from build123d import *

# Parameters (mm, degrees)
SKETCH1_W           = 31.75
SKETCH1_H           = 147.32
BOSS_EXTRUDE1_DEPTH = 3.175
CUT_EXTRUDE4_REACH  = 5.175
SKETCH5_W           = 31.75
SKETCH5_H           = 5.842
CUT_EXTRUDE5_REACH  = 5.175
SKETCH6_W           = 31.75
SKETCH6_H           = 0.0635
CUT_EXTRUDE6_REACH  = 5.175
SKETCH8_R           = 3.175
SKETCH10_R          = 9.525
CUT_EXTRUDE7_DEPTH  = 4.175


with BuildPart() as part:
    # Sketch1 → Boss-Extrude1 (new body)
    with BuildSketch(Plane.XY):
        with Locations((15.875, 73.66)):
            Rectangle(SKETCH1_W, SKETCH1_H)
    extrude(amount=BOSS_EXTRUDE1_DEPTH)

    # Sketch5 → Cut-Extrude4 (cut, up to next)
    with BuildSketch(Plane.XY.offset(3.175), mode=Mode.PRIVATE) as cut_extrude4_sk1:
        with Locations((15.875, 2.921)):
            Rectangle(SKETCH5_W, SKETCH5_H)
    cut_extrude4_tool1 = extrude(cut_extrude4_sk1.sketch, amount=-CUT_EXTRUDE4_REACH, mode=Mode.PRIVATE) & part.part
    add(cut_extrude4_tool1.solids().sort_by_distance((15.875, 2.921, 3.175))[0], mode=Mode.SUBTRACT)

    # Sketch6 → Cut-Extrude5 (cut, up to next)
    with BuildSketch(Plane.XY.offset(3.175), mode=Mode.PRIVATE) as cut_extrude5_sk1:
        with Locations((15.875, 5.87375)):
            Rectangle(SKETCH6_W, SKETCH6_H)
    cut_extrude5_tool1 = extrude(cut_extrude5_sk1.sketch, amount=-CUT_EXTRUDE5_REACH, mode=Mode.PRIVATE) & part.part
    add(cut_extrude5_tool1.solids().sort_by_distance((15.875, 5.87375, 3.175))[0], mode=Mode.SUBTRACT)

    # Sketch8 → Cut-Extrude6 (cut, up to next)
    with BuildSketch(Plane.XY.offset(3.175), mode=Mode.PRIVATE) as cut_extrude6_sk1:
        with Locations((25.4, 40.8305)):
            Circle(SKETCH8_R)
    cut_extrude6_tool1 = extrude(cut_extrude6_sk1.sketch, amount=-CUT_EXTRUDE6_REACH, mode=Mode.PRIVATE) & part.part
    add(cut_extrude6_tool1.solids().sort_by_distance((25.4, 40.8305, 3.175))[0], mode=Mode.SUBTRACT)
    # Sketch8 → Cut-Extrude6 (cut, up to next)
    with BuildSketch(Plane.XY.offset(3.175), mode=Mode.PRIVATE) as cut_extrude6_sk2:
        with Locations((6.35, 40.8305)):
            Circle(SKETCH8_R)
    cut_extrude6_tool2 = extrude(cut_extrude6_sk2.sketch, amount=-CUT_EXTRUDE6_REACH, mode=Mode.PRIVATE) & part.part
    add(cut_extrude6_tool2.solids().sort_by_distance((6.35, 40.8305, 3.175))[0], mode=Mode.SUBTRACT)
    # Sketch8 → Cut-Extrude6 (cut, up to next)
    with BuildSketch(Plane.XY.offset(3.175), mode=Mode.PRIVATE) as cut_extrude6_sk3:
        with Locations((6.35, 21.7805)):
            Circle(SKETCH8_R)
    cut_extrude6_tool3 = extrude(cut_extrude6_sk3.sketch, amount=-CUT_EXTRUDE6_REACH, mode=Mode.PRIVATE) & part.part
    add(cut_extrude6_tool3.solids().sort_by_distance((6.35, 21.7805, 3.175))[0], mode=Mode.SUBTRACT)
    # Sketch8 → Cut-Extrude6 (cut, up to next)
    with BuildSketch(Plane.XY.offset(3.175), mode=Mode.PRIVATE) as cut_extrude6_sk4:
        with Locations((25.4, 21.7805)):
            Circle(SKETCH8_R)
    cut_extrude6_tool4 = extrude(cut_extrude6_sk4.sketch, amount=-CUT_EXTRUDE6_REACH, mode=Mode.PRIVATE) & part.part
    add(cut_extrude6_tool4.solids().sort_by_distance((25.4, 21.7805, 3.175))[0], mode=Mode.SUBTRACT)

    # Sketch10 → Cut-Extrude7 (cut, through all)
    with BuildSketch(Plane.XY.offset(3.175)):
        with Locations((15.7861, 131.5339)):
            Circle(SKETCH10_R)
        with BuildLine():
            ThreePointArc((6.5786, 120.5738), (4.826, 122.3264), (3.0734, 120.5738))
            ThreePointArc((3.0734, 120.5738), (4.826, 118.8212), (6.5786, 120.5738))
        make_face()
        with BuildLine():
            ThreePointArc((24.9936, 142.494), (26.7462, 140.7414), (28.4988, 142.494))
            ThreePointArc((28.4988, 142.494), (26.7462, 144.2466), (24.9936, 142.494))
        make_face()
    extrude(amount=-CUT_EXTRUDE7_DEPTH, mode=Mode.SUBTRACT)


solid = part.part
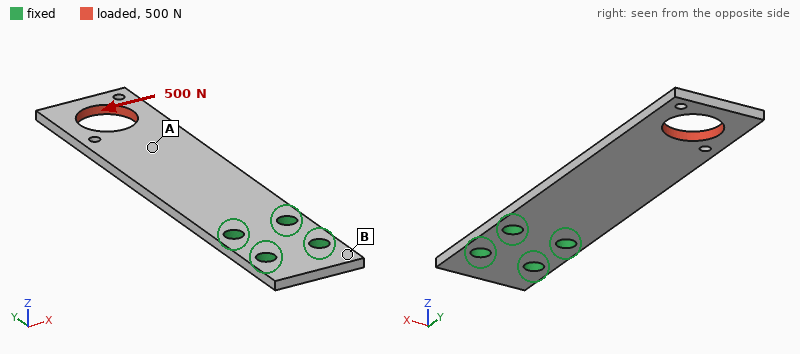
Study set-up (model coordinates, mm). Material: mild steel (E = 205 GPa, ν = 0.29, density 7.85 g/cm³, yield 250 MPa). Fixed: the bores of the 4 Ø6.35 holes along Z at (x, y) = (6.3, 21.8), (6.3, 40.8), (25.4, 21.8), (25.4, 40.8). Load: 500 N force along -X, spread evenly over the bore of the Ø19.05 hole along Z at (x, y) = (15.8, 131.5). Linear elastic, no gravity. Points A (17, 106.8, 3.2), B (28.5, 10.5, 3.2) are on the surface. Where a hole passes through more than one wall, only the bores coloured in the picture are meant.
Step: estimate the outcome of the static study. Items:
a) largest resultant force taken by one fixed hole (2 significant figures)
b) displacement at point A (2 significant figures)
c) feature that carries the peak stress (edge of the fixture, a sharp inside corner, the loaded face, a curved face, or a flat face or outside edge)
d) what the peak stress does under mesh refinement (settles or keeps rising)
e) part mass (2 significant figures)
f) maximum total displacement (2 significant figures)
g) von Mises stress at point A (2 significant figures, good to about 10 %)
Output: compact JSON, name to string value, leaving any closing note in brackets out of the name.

{"largest resultant force taken by one fixed hole": "2.0 kN", "displacement at point A": "0.046 mm", "feature that carries the peak stress": "edge of the fixture", "what the peak stress does under mesh refinement": "keeps rising", "part mass": "100 g", "maximum total displacement": "0.10 mm", "von Mises stress at point A": "15 MPa"}
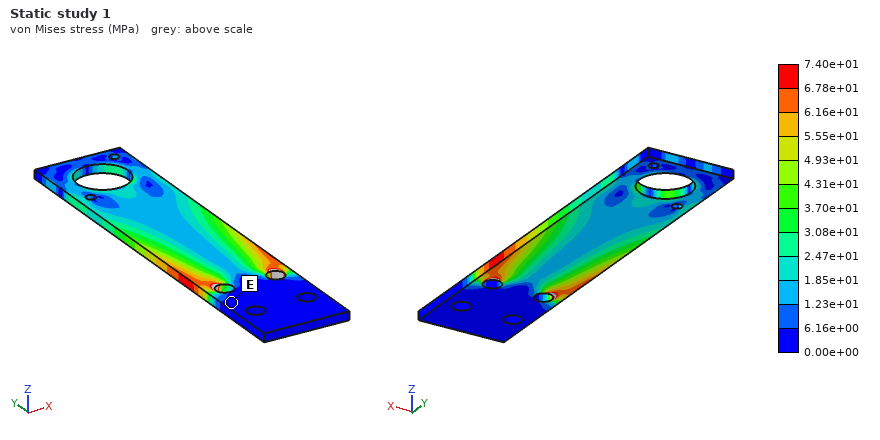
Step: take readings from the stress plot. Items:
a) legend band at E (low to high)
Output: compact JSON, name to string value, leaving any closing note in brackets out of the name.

{"legend band at E": "0.00e+00 to 6.16e+00 MPa"}
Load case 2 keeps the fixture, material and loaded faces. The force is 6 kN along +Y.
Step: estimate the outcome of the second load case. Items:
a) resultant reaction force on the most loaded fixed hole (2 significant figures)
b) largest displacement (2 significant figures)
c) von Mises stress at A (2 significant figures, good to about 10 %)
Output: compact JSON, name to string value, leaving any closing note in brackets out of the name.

{"resultant reaction force on the most loaded fixed hole": "2.9 kN", "largest displacement": "45 µm", "von Mises stress at A": "45 MPa"}
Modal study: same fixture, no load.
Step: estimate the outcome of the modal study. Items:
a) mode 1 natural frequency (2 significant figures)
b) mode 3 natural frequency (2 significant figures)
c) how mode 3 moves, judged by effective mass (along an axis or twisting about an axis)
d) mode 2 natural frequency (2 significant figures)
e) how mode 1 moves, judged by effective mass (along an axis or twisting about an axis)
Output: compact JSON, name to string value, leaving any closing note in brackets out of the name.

{"mode 1 natural frequency": "280 Hz", "mode 3 natural frequency": "1600 Hz", "how mode 3 moves, judged by effective mass": "twisting about Y", "mode 2 natural frequency": "1500 Hz", "how mode 1 moves, judged by effective mass": "along Z"}
